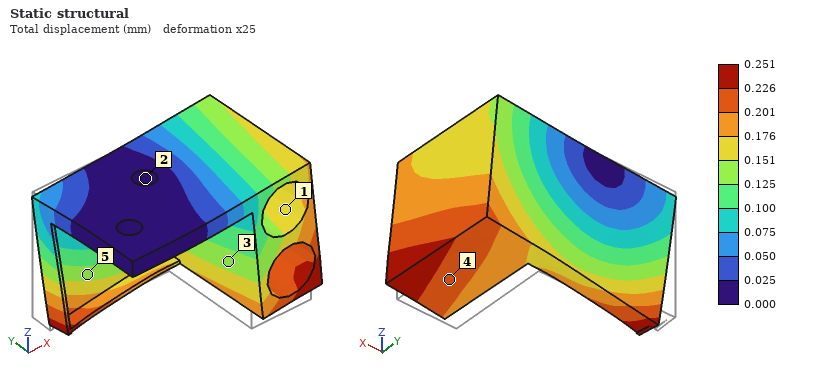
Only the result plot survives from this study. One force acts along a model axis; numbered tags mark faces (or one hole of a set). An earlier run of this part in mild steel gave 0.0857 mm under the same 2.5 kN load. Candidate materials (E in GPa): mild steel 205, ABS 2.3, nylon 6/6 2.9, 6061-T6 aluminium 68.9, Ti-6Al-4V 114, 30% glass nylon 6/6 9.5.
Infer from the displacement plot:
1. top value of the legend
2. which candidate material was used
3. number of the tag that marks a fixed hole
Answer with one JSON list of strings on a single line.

["0.251 mm", "6061-T6 aluminium", "2"]
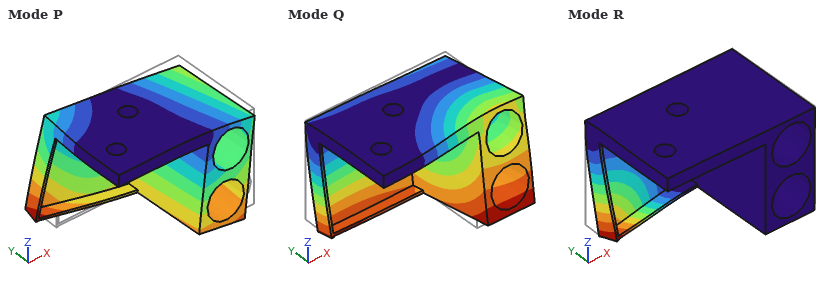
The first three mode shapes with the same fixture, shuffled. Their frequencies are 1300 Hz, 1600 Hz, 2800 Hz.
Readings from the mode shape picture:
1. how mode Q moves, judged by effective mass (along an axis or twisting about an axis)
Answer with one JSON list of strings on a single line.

["along Y"]
